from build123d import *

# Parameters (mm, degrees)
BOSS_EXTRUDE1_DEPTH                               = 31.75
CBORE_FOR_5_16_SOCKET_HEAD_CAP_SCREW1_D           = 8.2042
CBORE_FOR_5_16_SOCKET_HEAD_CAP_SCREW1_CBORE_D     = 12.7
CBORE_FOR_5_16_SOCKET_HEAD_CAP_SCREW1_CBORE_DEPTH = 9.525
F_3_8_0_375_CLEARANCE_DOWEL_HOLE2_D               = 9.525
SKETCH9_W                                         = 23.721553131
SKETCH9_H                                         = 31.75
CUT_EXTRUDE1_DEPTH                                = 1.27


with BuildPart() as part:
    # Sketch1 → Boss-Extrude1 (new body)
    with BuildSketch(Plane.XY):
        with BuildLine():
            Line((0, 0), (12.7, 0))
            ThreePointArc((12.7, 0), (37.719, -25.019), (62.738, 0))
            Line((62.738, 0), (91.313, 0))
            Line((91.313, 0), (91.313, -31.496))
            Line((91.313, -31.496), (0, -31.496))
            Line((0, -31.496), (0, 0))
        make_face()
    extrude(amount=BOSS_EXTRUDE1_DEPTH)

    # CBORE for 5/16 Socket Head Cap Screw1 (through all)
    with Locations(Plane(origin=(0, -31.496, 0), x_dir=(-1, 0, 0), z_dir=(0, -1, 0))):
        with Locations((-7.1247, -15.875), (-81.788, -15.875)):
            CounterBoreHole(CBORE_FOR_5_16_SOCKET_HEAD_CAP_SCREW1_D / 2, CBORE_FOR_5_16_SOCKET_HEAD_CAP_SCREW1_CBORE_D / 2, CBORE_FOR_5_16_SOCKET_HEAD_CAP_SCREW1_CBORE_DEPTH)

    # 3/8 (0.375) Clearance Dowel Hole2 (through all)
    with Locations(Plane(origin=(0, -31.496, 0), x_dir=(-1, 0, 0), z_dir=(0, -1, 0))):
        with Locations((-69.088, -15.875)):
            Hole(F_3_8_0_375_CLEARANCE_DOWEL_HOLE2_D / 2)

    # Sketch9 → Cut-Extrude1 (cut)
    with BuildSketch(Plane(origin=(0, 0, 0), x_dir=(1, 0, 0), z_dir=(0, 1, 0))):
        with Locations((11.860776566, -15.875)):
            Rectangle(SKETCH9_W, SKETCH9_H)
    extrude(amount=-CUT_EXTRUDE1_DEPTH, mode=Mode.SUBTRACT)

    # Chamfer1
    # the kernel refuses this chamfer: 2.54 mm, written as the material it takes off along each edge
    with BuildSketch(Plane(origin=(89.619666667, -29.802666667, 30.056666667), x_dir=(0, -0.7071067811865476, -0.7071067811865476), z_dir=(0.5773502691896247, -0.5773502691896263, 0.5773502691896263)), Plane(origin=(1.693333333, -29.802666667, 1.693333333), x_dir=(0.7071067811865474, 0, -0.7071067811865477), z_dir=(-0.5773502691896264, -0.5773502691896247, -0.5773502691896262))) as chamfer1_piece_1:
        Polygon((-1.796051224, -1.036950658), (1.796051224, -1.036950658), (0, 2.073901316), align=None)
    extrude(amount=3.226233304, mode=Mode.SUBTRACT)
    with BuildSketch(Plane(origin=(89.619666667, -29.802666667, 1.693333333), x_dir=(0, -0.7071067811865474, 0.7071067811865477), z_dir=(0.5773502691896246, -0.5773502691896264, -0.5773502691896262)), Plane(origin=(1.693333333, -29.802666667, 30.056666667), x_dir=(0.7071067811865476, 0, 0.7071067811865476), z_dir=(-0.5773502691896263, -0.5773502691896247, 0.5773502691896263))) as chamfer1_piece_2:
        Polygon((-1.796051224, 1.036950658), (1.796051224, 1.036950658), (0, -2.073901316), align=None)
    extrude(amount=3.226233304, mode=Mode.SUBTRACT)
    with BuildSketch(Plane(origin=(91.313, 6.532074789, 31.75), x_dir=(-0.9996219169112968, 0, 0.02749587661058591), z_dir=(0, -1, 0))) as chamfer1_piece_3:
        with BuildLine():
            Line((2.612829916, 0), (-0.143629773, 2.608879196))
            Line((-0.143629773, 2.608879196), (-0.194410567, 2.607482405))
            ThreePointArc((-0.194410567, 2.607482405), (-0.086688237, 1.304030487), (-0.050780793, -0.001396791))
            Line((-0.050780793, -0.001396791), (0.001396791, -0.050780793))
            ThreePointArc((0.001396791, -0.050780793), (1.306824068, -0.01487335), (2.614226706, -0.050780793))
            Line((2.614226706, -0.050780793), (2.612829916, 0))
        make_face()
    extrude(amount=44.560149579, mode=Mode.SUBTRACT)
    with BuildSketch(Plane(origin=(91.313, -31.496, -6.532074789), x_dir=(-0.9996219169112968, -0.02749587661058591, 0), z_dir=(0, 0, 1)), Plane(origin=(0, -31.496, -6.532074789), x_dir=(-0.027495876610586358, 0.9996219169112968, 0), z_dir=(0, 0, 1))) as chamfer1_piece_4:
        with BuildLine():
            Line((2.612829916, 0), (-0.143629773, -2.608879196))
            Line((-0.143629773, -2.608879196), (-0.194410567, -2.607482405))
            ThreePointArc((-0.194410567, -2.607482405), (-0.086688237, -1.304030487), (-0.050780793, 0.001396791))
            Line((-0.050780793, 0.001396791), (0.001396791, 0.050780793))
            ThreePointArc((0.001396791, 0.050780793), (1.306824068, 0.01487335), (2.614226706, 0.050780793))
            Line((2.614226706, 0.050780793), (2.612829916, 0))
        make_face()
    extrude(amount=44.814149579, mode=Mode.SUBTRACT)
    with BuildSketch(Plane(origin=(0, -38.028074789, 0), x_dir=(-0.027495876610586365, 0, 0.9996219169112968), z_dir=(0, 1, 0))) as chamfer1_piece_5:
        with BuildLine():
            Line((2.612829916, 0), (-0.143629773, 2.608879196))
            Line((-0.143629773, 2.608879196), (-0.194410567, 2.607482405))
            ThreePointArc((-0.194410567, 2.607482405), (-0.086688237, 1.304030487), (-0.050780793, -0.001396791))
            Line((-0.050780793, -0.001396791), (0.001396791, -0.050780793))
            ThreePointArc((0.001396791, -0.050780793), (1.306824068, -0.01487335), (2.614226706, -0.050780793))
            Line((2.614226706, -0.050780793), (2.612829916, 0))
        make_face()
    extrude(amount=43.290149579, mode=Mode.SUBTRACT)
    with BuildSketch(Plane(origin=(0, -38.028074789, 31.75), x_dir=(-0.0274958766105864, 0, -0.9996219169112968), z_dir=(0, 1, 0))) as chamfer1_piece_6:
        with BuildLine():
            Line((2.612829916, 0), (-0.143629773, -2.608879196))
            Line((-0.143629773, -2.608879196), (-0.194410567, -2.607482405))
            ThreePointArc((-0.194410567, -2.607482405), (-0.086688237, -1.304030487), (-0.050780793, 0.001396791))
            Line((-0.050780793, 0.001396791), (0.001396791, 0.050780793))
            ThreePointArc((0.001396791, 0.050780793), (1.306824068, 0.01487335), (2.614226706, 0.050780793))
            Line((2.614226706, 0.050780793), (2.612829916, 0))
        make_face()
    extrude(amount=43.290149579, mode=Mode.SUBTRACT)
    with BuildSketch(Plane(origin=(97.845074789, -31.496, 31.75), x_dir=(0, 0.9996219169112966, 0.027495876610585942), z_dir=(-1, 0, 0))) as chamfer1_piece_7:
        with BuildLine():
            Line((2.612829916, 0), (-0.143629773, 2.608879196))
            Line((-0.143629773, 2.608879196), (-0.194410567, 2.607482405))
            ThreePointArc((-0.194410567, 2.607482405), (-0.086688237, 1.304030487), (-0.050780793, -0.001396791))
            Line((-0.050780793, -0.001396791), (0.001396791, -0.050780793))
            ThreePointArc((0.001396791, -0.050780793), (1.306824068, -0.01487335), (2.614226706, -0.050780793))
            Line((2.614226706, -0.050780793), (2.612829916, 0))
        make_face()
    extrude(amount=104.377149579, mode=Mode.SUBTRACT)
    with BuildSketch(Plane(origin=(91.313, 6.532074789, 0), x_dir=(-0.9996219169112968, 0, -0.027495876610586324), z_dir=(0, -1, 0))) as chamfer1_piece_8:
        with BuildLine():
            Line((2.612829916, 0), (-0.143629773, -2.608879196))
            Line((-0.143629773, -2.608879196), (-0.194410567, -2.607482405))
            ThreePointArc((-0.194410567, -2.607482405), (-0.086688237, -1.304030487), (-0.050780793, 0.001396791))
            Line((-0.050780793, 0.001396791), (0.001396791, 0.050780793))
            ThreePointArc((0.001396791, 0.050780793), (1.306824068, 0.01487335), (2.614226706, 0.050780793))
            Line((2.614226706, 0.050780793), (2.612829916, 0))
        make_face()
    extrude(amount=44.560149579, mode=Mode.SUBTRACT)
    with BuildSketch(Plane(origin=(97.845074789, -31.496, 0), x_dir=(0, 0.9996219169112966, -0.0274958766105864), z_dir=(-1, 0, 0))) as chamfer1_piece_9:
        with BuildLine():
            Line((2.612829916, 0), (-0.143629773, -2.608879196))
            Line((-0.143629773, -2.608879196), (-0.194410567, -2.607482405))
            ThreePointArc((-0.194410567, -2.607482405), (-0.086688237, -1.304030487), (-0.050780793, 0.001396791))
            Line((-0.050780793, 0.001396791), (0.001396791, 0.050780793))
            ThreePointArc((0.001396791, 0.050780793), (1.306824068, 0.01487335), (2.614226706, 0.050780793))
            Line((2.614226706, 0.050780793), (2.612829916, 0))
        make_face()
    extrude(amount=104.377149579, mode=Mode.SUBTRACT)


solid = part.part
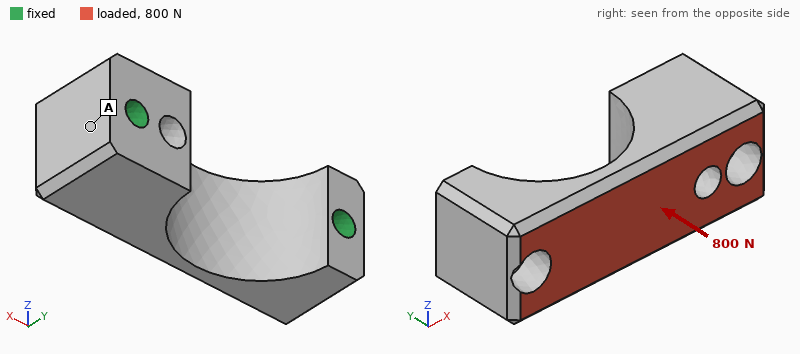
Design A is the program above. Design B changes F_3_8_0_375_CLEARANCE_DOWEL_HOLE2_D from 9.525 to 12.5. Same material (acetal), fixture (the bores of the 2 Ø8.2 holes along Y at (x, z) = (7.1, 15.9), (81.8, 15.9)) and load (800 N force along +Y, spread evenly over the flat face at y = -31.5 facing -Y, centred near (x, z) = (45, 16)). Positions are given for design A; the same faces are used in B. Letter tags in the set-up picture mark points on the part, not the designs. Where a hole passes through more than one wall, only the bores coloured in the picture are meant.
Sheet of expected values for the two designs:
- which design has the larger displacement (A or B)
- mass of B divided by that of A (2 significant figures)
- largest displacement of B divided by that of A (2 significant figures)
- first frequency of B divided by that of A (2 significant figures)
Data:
B
0.97
1.1
0.97
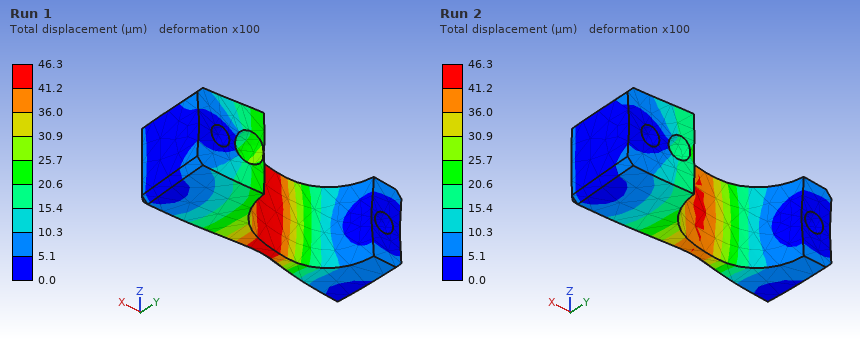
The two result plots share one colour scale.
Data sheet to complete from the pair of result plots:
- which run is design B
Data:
Run 1
